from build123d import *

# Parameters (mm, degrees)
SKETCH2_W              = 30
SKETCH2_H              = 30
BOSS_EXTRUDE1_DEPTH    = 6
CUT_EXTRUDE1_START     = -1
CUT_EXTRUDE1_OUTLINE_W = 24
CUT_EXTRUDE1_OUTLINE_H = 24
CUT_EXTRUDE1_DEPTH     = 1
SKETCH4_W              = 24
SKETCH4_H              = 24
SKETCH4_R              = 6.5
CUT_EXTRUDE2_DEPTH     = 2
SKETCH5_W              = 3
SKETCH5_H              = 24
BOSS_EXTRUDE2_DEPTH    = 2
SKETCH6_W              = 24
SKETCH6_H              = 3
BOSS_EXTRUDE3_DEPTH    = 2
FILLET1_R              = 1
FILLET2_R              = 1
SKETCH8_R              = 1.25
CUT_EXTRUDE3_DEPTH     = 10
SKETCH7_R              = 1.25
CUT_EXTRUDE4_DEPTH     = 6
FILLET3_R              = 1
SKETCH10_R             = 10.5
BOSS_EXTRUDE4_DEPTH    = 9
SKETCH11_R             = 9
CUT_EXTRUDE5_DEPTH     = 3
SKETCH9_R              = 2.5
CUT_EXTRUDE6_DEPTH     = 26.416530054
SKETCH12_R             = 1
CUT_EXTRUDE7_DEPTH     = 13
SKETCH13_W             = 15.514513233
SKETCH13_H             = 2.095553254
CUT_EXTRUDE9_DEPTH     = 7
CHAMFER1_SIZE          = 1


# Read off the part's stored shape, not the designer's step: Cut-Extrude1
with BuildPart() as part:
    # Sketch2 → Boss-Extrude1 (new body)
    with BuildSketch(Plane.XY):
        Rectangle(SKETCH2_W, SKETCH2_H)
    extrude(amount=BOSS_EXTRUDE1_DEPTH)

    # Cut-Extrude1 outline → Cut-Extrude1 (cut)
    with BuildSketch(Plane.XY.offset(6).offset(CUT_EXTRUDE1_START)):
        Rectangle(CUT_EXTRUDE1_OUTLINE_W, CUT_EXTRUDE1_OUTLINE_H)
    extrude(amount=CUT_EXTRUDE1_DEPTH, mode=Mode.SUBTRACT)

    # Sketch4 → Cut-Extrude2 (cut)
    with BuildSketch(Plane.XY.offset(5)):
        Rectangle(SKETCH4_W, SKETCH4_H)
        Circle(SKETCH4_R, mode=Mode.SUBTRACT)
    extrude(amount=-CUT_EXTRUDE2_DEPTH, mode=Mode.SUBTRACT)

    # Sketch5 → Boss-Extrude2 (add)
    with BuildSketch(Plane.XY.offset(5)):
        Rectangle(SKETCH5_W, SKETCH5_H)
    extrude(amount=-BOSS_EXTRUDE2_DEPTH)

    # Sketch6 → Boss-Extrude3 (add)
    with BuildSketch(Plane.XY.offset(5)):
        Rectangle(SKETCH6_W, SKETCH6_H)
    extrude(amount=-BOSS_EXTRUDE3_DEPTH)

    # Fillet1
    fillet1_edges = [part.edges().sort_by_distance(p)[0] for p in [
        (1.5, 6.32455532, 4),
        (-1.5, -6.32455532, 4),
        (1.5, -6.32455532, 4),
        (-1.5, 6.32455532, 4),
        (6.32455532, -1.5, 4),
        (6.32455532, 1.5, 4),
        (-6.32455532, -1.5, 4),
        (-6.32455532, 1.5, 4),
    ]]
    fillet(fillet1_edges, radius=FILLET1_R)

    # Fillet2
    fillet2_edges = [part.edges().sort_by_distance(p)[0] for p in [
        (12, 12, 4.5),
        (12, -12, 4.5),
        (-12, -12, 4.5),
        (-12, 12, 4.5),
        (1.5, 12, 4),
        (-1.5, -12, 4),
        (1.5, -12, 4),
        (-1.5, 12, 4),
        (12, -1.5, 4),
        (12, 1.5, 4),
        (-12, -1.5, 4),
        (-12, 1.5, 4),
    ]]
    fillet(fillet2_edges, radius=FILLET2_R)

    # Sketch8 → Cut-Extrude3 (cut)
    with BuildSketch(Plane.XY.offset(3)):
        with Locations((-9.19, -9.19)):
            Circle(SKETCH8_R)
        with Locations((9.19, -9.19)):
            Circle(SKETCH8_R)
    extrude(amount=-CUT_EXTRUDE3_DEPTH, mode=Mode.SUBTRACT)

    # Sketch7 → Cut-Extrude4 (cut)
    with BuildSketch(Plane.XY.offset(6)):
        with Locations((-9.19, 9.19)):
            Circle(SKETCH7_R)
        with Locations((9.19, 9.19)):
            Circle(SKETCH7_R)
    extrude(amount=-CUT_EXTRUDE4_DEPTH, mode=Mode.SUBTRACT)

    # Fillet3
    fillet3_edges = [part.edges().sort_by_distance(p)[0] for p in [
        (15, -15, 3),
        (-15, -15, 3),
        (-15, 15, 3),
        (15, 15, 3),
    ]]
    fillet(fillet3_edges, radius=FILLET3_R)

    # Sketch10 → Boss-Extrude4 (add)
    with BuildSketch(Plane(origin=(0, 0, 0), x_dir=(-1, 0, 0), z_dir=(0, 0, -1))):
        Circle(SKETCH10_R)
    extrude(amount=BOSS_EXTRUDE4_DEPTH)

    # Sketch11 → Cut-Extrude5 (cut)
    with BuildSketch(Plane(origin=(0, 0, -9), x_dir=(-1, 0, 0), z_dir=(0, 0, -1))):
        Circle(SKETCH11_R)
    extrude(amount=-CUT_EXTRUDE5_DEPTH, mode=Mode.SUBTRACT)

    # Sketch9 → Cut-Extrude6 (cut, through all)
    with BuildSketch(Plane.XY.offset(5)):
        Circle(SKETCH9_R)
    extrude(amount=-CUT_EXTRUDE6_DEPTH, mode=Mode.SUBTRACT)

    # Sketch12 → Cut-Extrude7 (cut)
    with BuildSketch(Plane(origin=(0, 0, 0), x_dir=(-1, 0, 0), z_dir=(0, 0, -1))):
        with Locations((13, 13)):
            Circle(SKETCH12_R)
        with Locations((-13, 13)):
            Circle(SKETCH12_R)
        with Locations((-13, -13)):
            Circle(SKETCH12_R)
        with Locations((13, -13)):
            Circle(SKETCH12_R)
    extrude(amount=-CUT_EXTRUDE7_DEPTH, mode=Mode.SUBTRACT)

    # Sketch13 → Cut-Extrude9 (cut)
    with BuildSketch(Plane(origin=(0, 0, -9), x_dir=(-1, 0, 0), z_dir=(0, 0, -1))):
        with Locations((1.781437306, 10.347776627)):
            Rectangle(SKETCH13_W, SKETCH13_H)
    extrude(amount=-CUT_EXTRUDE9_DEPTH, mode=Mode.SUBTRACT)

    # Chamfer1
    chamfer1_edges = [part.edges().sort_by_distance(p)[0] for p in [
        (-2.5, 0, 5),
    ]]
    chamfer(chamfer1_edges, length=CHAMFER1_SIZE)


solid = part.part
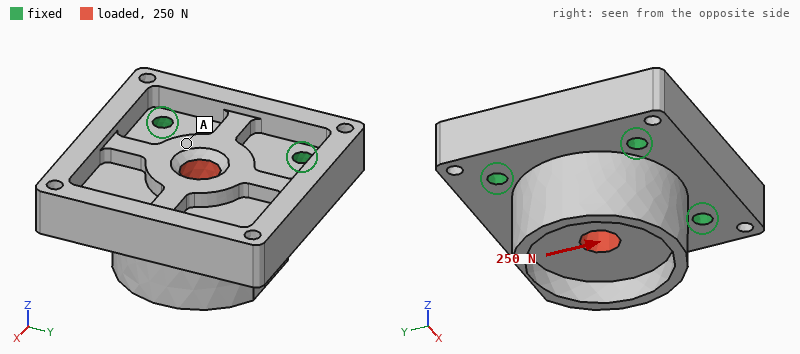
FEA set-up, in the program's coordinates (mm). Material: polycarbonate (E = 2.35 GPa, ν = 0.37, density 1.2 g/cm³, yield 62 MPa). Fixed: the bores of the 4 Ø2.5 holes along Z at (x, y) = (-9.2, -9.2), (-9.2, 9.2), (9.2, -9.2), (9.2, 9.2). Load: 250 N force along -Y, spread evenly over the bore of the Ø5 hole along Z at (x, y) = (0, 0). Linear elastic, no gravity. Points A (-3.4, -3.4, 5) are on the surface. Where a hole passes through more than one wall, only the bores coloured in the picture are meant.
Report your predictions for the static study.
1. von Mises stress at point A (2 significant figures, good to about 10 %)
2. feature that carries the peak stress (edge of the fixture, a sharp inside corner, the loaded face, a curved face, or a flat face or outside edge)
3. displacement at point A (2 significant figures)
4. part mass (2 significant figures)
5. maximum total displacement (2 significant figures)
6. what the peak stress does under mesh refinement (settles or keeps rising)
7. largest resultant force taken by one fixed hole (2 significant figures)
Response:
0.66 MPa
edge of the fixture
8.0 µm
7.2 g
15 µm
keeps rising
68 N
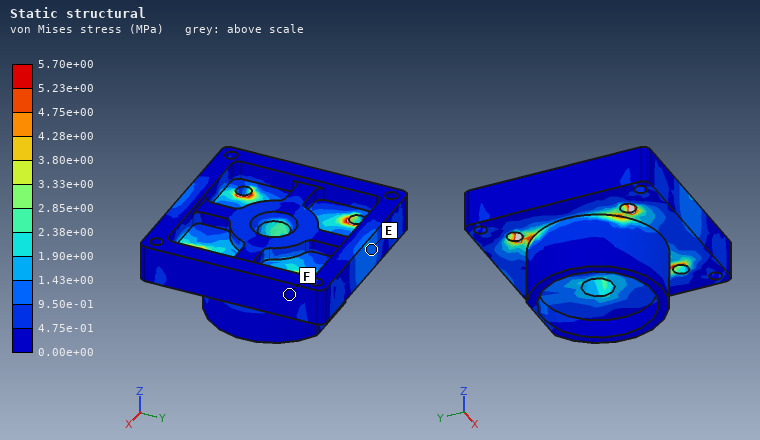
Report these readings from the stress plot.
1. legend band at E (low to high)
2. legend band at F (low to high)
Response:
9.50e-01 to 1.43e+00 MPa
0.00e+00 to 4.75e-01 MPa
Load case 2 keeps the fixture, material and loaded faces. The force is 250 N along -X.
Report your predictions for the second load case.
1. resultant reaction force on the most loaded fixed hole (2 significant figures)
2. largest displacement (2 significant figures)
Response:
68 N
15 µm
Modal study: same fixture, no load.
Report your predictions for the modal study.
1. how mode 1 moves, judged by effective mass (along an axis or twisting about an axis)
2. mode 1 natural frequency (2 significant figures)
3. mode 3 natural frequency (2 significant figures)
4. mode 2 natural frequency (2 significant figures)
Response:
along Z
9000 Hz
9700 Hz
9600 Hz
